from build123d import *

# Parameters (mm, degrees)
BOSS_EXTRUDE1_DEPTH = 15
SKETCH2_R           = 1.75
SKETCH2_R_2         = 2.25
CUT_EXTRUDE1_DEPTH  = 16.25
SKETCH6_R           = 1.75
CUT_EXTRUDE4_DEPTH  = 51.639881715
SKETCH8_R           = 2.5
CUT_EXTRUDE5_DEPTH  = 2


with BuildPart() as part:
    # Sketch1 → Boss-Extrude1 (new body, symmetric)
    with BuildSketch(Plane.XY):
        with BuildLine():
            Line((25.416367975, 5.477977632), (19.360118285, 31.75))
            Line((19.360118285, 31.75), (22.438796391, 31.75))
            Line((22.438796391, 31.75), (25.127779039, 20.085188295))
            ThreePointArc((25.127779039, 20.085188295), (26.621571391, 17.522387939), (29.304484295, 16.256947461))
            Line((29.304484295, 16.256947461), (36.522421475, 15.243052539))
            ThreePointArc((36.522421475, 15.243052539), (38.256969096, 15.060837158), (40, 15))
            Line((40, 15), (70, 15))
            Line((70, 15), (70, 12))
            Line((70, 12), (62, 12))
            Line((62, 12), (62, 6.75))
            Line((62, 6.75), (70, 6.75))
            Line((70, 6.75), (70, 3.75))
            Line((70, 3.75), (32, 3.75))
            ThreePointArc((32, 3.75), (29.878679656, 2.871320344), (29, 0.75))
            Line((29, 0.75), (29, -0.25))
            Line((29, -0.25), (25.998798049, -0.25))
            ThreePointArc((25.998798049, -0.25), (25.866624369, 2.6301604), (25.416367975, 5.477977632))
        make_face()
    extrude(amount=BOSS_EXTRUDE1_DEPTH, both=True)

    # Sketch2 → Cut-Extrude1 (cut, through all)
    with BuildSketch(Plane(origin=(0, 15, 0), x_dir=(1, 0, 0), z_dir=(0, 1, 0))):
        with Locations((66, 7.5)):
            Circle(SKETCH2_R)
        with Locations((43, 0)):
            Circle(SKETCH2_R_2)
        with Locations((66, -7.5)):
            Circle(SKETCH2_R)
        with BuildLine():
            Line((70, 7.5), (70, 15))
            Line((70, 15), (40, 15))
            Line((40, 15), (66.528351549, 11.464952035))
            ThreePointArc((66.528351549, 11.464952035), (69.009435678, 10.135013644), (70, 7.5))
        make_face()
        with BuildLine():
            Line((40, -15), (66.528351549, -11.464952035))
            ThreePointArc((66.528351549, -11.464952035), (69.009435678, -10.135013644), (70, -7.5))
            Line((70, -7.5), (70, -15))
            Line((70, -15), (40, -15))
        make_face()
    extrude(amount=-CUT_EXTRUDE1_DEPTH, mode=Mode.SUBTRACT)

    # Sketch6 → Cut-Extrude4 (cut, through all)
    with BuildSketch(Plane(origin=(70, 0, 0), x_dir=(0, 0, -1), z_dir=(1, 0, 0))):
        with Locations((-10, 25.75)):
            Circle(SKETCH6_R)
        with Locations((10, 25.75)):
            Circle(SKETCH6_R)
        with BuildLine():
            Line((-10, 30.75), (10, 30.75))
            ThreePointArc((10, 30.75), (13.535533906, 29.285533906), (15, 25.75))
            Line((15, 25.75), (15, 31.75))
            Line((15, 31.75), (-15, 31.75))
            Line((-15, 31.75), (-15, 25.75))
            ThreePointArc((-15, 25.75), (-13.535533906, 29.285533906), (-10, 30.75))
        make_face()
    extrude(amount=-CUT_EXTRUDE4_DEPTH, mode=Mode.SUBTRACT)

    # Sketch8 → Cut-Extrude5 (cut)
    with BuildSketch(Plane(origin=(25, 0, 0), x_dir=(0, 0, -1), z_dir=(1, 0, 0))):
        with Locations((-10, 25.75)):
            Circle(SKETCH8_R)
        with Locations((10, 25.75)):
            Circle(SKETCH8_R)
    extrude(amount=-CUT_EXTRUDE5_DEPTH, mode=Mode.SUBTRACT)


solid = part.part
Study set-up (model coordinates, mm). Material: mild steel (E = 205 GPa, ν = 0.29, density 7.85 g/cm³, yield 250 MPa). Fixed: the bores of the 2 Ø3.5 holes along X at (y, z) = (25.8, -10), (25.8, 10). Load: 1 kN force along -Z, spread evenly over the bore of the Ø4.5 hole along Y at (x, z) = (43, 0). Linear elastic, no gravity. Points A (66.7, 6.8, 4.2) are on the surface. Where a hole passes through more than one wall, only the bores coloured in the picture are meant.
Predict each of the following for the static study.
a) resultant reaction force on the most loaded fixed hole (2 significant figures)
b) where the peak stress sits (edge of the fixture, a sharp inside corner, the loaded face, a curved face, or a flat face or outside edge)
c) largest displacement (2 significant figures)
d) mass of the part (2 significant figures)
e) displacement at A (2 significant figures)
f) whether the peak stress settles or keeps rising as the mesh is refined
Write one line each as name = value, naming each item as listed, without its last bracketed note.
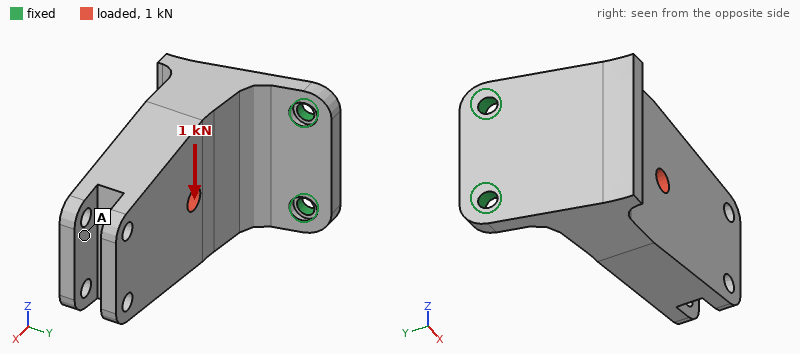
resultant reaction force on the most loaded fixed hole = 1.3 kN
where the peak stress sits = edge of the fixture
largest displacement = 79 µm
mass of the part = 120 g
displacement at A = 69 µm
whether the peak stress settles or keeps rising as the mesh is refined = keeps rising
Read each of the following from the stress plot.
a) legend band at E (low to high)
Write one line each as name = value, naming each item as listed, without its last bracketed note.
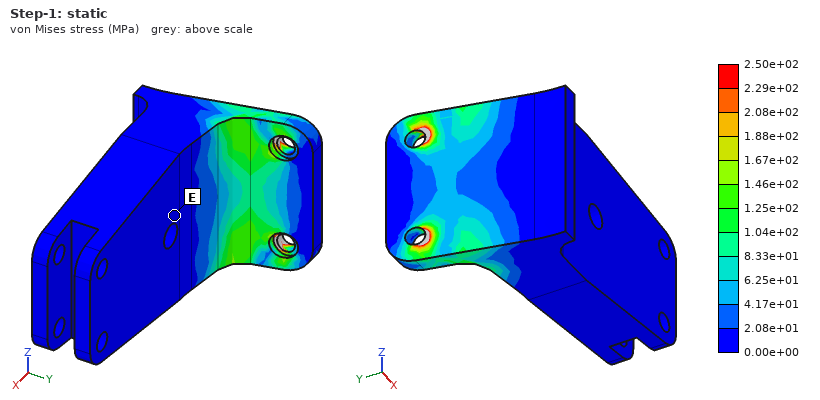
legend band at E = 0.00e+00 to 2.08e+01 MPa
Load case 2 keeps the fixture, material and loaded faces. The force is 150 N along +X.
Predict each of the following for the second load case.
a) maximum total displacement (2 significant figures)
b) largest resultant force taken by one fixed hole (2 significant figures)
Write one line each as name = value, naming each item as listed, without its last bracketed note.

maximum total displacement = 79 µm
largest resultant force taken by one fixed hole = 75 N
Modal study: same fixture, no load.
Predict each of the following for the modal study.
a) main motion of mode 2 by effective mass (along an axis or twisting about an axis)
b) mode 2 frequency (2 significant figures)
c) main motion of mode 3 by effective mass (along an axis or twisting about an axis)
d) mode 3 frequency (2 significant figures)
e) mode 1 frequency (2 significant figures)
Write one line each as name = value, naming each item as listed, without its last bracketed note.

main motion of mode 2 by effective mass = along Z
mode 2 frequency = 2100 Hz
main motion of mode 3 by effective mass = along X
mode 3 frequency = 5600 Hz
mode 1 frequency = 620 Hz
